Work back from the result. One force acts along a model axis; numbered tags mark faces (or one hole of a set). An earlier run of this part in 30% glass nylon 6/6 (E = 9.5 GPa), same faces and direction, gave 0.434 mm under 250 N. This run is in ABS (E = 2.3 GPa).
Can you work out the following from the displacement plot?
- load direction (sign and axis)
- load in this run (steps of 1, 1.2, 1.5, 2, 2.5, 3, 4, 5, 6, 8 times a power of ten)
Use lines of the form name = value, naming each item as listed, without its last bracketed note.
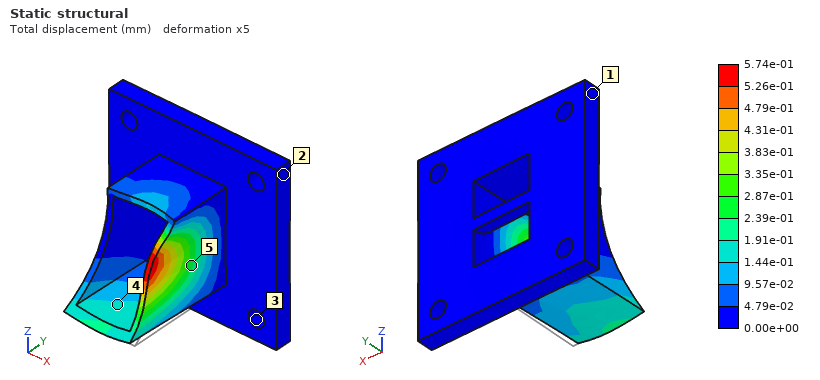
load direction = -X
load in this run = 80 N
